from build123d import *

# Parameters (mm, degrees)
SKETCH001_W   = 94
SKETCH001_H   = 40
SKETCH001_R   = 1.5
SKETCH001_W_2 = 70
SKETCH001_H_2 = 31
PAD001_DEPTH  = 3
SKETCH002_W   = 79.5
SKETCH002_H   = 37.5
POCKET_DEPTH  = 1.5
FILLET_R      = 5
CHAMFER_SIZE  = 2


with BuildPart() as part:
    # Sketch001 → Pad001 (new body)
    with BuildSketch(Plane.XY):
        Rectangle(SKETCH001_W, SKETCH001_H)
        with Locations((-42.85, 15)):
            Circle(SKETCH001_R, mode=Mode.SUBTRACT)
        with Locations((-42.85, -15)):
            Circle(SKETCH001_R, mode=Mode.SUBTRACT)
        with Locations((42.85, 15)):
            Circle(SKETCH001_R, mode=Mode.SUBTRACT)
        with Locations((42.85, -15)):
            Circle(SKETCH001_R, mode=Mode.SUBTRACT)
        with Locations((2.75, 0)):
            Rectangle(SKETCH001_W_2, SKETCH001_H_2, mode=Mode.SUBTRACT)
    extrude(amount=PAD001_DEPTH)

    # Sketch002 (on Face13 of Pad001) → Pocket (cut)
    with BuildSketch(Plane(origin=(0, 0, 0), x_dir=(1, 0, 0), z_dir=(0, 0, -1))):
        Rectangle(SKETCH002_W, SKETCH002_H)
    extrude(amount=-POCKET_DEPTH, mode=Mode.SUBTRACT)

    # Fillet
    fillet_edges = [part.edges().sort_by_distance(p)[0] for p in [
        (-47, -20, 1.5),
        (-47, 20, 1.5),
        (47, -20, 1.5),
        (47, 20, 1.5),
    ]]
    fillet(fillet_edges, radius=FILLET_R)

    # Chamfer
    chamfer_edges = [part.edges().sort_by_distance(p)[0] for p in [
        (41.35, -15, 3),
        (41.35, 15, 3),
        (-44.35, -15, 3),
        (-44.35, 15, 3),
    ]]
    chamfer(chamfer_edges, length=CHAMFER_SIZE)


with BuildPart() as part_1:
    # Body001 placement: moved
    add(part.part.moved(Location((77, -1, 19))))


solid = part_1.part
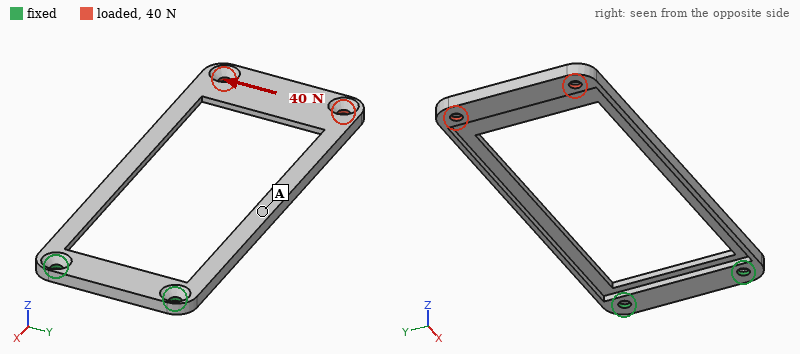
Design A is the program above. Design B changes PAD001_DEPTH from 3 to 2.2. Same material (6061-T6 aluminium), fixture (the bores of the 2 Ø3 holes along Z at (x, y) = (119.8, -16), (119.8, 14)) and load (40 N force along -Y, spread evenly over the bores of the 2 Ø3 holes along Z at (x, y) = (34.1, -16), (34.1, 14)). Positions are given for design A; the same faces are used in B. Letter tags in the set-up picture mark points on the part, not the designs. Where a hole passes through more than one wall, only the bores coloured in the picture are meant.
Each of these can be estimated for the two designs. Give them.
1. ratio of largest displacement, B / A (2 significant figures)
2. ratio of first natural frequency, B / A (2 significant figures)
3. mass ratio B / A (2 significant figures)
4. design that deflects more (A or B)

2.6
0.76
0.63
B
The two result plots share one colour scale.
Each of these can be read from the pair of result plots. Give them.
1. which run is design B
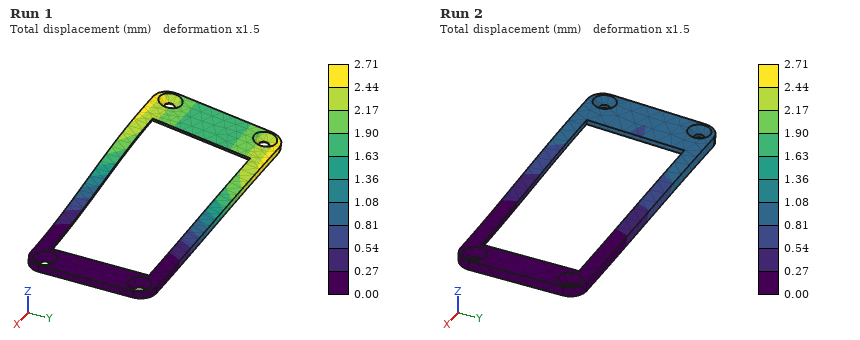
Run 1
